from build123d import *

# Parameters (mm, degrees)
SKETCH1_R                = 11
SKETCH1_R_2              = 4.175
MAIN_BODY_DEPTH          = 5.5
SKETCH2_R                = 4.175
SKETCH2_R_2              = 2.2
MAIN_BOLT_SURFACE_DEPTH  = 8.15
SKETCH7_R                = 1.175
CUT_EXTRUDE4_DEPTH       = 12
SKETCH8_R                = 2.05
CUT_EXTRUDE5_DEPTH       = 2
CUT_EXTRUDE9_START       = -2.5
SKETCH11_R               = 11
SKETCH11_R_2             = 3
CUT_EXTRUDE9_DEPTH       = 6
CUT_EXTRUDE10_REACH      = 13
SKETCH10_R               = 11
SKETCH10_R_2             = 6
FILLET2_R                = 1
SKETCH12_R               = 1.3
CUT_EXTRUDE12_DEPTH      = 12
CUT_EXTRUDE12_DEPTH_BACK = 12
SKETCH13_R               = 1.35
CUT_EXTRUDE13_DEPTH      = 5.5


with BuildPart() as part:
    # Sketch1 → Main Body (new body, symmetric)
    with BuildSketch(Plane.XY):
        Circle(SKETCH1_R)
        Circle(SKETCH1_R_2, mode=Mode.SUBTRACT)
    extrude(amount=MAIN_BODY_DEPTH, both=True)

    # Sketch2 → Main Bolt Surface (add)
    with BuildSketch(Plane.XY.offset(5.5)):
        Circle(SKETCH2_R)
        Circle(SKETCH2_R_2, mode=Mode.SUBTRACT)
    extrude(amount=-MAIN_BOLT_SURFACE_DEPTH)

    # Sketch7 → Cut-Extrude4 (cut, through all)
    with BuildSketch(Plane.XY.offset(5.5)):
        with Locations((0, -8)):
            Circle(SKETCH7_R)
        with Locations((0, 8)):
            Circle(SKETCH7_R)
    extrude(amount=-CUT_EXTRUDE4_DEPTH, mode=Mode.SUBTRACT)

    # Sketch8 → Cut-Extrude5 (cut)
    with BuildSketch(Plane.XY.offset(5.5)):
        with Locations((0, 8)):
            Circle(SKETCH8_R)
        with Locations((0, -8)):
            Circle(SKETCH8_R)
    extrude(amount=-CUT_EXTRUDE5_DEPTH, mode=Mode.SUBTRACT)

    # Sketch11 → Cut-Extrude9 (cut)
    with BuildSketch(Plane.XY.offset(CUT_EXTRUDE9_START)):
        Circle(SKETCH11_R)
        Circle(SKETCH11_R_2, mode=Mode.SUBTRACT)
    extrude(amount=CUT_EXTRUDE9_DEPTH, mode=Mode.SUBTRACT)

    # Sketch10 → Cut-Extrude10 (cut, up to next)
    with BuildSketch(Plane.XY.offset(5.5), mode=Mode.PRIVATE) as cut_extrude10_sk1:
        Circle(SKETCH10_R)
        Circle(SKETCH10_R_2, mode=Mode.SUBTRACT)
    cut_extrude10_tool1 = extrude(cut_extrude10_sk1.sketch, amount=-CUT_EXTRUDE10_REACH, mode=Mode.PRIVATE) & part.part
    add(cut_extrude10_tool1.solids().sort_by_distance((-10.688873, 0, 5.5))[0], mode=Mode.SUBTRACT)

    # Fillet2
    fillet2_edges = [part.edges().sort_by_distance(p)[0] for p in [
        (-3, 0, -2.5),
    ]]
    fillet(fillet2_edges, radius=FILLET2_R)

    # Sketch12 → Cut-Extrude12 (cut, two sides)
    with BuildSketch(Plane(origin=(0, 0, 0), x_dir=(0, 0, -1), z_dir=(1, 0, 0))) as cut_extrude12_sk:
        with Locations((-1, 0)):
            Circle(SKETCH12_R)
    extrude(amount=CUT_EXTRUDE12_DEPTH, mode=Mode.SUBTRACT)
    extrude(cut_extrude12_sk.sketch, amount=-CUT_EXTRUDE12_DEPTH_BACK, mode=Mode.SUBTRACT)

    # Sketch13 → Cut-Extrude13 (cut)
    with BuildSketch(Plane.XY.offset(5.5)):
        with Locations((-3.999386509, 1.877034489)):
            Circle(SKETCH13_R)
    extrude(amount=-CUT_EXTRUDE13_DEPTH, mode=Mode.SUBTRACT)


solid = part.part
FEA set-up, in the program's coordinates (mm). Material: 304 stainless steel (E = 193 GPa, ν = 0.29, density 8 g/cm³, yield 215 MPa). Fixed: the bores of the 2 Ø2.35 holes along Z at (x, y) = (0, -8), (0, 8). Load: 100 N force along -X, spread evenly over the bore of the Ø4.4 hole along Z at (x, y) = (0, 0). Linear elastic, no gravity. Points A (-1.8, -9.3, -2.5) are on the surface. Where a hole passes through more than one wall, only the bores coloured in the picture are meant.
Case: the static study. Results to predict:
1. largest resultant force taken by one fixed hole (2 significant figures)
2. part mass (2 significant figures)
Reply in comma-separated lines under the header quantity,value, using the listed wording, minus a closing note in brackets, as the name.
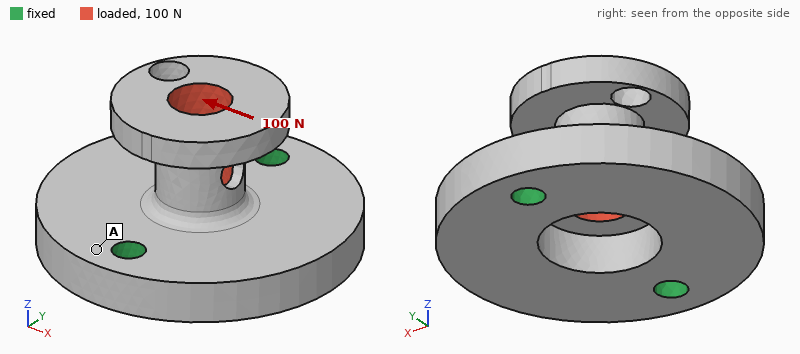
quantity,value
largest resultant force taken by one fixed hole,50 N
part mass,9.7 g
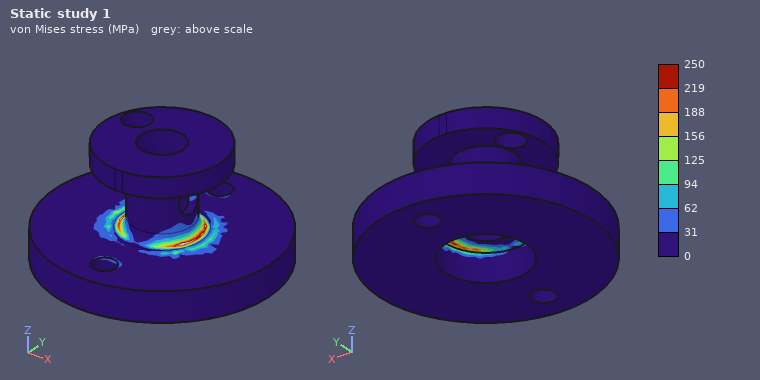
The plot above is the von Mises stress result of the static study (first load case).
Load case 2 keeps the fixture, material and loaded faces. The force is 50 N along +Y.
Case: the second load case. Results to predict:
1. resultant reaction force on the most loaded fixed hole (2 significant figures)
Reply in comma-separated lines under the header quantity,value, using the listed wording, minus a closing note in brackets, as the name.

quantity,value
resultant reaction force on the most loaded fixed hole,33 N
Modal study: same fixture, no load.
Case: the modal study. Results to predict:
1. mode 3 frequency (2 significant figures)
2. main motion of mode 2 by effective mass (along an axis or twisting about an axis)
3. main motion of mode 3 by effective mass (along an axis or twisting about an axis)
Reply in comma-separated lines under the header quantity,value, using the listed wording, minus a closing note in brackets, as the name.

quantity,value
mode 3 frequency,19 kHz
main motion of mode 2 by effective mass,along Y
main motion of mode 3 by effective mass,along Z
